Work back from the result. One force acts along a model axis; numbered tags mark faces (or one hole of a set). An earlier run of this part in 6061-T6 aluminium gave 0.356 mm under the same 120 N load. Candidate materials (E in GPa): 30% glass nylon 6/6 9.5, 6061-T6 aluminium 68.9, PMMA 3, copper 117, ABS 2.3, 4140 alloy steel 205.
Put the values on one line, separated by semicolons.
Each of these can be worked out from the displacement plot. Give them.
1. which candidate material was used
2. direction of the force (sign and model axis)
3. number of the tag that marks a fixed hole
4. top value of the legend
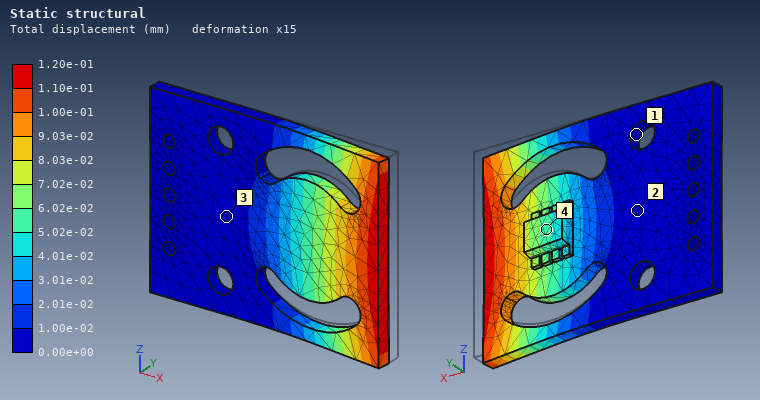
4140 alloy steel; -Y; 1; 1.20e-01 mm
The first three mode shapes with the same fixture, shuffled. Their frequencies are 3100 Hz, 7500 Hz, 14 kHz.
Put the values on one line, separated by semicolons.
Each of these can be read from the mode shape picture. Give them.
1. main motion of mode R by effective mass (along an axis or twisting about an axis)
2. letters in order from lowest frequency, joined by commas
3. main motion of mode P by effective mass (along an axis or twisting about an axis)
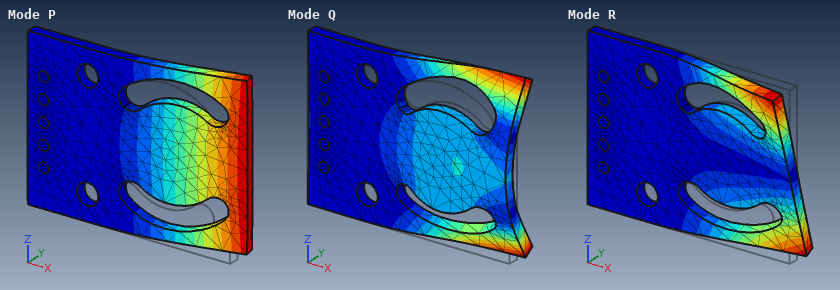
twisting about X; P, R, Q; along Y
